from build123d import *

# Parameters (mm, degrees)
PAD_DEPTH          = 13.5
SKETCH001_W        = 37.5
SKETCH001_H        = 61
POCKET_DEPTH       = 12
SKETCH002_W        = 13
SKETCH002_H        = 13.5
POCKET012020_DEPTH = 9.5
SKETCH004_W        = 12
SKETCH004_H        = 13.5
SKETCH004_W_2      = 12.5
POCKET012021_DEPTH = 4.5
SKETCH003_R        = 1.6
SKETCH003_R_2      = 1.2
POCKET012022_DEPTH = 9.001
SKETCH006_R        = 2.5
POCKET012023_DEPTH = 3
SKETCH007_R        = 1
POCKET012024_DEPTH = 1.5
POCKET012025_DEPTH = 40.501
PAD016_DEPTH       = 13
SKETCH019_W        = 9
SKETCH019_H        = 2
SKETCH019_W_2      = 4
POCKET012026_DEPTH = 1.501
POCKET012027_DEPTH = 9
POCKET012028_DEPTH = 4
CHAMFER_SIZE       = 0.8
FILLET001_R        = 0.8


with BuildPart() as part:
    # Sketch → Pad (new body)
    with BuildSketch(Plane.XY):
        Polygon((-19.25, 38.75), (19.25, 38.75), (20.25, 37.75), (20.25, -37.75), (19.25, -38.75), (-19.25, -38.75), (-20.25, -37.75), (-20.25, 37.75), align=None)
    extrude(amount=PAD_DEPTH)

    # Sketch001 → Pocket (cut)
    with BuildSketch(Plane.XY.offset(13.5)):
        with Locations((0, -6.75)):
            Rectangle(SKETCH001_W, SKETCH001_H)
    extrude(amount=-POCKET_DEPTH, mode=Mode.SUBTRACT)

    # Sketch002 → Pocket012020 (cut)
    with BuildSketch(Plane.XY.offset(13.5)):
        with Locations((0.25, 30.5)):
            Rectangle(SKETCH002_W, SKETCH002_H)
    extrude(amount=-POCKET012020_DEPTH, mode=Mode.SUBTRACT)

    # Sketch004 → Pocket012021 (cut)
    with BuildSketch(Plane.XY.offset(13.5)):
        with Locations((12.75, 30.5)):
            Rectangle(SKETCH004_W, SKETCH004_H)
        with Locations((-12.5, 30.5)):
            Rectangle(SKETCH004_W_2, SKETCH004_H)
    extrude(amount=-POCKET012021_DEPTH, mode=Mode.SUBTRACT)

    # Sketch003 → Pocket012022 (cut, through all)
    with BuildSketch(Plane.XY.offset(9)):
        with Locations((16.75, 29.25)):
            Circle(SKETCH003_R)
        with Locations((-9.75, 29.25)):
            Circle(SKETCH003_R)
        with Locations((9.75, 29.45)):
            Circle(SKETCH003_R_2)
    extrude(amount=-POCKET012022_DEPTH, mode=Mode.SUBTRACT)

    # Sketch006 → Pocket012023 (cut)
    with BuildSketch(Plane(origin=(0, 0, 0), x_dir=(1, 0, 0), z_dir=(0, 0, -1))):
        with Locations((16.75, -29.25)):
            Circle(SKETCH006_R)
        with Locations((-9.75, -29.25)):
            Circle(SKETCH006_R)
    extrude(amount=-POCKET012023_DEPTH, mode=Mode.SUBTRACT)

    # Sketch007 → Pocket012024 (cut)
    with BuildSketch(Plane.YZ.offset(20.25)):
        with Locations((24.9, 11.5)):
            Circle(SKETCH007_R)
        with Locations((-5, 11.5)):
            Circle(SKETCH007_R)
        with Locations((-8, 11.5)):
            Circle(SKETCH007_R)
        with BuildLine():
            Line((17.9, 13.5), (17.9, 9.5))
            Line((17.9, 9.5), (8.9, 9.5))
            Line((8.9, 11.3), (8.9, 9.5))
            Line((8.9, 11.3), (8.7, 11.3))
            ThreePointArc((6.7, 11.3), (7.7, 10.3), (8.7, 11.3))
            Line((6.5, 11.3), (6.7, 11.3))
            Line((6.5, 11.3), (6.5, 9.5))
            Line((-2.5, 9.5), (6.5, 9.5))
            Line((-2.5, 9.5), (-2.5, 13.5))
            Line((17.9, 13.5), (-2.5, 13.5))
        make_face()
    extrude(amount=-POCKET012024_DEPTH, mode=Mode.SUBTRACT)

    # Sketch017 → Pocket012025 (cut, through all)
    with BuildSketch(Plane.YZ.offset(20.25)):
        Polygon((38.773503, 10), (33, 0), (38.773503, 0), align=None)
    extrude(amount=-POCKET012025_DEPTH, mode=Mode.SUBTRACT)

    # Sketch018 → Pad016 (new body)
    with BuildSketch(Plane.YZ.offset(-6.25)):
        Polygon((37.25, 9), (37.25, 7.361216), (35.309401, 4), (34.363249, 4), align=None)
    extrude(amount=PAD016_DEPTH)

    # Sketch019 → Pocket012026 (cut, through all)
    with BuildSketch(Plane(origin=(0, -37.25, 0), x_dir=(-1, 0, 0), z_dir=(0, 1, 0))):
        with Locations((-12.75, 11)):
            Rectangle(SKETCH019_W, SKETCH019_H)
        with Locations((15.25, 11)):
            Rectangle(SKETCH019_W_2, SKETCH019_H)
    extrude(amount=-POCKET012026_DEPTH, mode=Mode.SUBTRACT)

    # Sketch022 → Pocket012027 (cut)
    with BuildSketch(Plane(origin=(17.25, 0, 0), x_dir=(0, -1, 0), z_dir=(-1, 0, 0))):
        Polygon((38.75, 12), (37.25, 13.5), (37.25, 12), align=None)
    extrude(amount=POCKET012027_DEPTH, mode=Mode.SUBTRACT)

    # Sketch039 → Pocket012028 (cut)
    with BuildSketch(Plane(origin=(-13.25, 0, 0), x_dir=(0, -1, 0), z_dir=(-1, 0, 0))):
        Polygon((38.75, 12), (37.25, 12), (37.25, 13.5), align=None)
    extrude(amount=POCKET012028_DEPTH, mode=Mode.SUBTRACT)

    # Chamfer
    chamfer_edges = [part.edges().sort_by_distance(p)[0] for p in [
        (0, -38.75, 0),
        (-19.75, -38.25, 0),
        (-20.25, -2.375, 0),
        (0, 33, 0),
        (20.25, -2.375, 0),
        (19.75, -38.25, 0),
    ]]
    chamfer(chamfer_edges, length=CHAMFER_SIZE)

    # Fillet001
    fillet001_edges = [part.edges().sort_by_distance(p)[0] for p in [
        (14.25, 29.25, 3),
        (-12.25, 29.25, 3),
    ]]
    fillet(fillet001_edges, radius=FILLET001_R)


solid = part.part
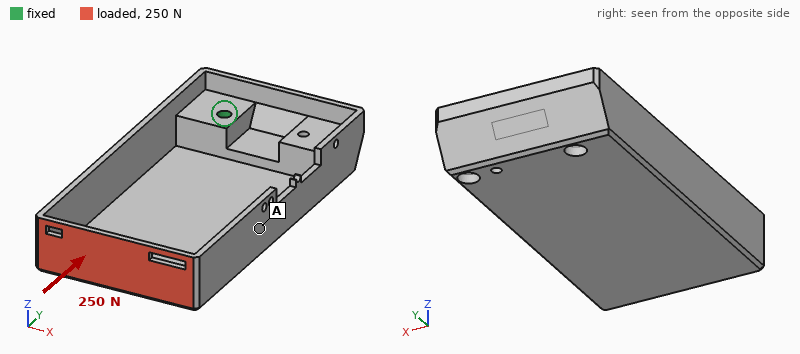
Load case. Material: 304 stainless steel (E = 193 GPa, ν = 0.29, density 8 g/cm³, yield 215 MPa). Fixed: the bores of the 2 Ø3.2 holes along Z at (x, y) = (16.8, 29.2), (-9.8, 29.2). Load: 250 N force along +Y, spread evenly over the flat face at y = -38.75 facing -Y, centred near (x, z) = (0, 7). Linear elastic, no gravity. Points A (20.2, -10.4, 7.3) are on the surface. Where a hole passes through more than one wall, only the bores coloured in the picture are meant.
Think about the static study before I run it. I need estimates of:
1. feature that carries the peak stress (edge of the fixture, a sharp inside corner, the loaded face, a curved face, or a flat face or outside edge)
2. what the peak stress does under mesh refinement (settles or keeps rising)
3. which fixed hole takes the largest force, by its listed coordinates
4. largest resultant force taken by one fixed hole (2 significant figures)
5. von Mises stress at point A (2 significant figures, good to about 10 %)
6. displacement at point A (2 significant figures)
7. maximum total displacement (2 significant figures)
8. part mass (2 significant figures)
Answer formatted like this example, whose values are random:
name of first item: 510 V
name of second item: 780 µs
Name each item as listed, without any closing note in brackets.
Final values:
feature that carries the peak stress: a sharp inside corner
what the peak stress does under mesh refinement: keeps rising
which fixed hole takes the largest force, by its listed coordinates: (-9.8, 29.2)
largest resultant force taken by one fixed hole: 150 N
von Mises stress at point A: 7.7 MPa
displacement at point A: 7.6 µm
maximum total displacement: 46 µm
part mass: 81 g
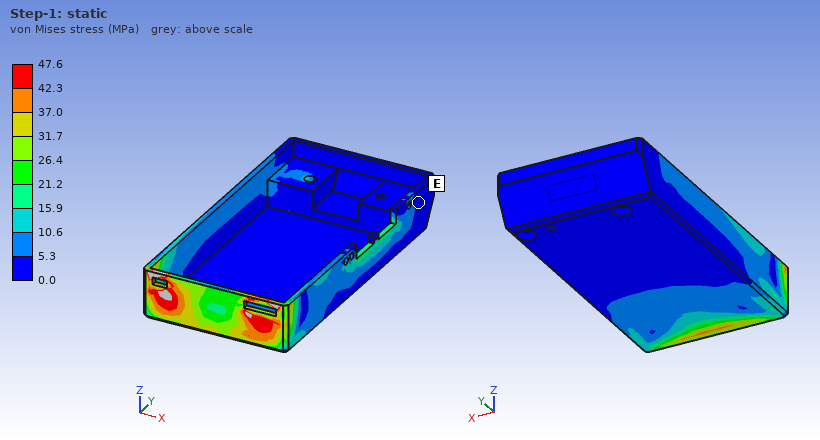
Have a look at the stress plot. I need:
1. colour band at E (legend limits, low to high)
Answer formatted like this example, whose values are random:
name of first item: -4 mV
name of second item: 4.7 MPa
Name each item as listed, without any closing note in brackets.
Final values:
colour band at E: 0.0 to 5.3 MPa
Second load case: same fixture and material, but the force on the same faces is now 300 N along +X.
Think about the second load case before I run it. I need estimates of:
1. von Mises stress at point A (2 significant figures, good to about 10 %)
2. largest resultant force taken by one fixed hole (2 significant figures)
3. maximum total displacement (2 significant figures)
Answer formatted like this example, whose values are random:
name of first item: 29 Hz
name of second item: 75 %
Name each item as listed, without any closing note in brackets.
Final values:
von Mises stress at point A: 26 MPa
largest resultant force taken by one fixed hole: 710 N
maximum total displacement: 0.17 mm
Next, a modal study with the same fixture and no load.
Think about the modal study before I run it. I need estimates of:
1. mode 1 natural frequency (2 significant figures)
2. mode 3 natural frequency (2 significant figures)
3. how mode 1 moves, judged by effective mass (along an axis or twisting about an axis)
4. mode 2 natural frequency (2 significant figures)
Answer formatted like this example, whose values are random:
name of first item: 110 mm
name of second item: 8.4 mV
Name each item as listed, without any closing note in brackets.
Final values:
mode 1 natural frequency: 1300 Hz
mode 3 natural frequency: 3800 Hz
how mode 1 moves, judged by effective mass: along Z
mode 2 natural frequency: 1600 Hz
